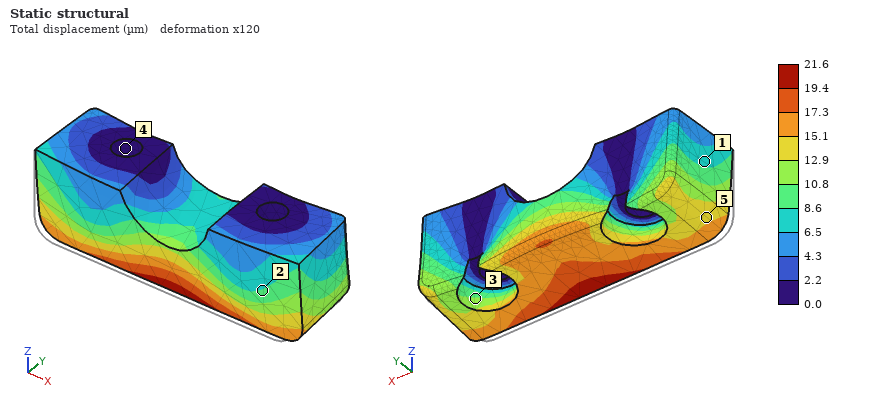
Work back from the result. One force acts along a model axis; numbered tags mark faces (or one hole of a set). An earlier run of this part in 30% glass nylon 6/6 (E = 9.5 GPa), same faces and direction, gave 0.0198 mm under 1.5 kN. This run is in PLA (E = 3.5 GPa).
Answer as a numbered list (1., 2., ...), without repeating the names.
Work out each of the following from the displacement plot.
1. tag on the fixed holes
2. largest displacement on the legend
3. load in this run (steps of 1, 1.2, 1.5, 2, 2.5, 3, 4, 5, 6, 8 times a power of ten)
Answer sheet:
1. 4
2. 21.6 µm
3. 600 N
